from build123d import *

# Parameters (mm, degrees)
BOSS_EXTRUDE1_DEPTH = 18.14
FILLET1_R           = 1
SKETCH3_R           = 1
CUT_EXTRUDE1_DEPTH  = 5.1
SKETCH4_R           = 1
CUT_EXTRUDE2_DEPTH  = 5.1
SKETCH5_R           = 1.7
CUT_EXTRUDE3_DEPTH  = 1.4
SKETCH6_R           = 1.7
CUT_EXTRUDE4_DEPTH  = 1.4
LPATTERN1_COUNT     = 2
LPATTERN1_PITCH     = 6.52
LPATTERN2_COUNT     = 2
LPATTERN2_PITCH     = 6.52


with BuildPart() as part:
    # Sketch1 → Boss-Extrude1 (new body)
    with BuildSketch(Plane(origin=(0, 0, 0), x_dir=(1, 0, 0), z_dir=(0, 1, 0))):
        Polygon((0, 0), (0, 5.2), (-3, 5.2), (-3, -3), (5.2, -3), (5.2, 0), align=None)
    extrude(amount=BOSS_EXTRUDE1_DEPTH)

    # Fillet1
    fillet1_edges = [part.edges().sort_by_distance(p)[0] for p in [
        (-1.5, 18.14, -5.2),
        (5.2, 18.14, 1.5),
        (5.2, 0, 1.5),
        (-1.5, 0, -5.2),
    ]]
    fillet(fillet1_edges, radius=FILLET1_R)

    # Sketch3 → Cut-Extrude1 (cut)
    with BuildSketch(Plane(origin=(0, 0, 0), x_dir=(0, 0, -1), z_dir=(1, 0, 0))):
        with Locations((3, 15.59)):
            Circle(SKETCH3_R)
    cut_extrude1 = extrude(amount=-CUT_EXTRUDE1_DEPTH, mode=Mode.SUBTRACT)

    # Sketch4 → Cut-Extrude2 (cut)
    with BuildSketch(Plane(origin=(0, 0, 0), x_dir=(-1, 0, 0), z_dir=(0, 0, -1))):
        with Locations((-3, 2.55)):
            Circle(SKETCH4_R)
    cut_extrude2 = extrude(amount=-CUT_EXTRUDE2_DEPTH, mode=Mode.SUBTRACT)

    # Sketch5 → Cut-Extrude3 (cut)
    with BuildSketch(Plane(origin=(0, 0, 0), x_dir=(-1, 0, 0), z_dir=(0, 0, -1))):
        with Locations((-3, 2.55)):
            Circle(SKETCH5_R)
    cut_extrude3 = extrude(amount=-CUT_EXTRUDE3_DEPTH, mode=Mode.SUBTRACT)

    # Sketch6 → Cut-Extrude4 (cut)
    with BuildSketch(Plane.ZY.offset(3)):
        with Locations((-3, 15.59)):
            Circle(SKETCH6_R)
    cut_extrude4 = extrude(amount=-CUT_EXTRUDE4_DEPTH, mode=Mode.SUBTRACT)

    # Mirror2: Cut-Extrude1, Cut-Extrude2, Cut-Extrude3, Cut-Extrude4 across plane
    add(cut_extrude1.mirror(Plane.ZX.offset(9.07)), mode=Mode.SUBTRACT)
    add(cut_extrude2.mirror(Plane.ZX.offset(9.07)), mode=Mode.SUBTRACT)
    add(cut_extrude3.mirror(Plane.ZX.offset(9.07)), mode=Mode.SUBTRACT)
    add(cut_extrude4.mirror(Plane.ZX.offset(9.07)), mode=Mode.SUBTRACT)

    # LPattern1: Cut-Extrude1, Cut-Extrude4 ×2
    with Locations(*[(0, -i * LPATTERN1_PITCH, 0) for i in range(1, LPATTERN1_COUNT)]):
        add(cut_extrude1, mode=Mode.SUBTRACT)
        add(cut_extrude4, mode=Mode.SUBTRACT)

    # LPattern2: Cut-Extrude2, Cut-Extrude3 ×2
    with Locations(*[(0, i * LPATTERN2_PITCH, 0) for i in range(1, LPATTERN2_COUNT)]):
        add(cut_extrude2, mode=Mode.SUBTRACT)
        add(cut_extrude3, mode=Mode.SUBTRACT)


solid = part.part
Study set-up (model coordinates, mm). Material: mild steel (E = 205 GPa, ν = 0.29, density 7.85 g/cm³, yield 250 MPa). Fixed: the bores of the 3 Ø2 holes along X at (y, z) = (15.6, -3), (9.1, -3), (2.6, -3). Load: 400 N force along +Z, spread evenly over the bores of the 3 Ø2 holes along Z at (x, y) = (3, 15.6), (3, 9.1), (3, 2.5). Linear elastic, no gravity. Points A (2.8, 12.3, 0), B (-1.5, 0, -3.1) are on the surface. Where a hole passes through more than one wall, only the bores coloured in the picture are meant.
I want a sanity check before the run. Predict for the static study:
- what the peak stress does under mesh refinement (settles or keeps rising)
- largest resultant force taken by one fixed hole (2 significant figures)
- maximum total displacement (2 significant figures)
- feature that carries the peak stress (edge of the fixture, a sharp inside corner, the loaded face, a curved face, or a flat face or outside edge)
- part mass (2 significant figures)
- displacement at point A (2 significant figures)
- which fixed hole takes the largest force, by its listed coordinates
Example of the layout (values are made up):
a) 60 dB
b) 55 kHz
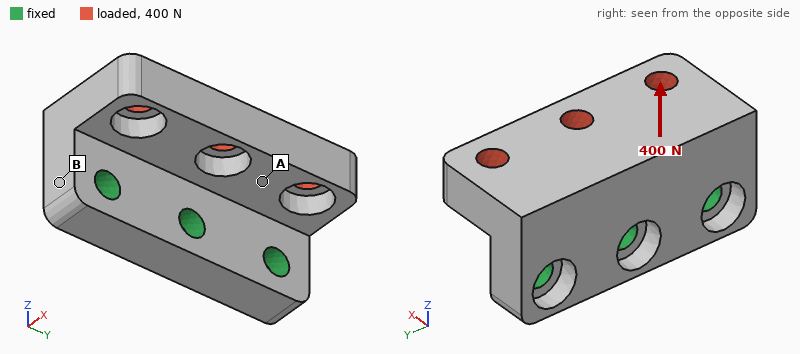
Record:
a) keeps rising
b) 150 N
c) 13 µm
d) edge of the fixture
e) 4.9 g
f) 6.6 µm
g) (9.1, -3)
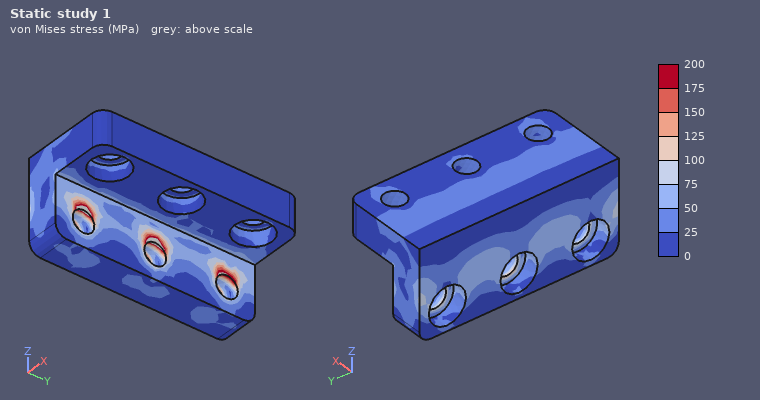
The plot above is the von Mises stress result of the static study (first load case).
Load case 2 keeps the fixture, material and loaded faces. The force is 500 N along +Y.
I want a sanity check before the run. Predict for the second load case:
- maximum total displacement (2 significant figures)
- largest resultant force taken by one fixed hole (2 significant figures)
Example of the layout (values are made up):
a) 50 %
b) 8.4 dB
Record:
a) 4.7 µm
b) 260 N
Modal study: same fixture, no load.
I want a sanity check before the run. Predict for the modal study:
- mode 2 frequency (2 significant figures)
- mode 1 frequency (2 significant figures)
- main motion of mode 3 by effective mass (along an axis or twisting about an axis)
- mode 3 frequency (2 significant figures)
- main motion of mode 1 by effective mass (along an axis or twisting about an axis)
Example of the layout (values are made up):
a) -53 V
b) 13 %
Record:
a) 34 kHz
b) 21 kHz
c) along Y
d) 57 kHz
e) along X
